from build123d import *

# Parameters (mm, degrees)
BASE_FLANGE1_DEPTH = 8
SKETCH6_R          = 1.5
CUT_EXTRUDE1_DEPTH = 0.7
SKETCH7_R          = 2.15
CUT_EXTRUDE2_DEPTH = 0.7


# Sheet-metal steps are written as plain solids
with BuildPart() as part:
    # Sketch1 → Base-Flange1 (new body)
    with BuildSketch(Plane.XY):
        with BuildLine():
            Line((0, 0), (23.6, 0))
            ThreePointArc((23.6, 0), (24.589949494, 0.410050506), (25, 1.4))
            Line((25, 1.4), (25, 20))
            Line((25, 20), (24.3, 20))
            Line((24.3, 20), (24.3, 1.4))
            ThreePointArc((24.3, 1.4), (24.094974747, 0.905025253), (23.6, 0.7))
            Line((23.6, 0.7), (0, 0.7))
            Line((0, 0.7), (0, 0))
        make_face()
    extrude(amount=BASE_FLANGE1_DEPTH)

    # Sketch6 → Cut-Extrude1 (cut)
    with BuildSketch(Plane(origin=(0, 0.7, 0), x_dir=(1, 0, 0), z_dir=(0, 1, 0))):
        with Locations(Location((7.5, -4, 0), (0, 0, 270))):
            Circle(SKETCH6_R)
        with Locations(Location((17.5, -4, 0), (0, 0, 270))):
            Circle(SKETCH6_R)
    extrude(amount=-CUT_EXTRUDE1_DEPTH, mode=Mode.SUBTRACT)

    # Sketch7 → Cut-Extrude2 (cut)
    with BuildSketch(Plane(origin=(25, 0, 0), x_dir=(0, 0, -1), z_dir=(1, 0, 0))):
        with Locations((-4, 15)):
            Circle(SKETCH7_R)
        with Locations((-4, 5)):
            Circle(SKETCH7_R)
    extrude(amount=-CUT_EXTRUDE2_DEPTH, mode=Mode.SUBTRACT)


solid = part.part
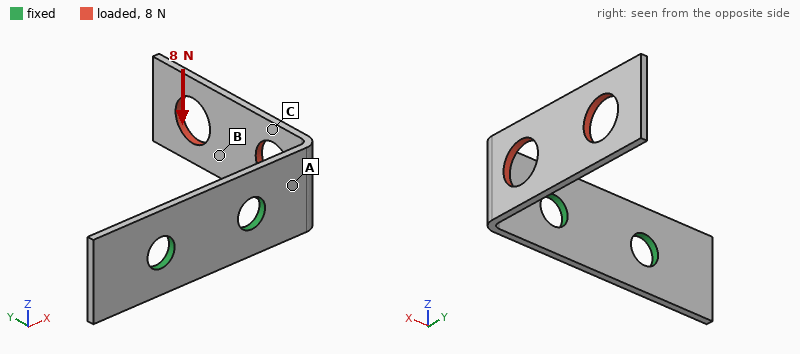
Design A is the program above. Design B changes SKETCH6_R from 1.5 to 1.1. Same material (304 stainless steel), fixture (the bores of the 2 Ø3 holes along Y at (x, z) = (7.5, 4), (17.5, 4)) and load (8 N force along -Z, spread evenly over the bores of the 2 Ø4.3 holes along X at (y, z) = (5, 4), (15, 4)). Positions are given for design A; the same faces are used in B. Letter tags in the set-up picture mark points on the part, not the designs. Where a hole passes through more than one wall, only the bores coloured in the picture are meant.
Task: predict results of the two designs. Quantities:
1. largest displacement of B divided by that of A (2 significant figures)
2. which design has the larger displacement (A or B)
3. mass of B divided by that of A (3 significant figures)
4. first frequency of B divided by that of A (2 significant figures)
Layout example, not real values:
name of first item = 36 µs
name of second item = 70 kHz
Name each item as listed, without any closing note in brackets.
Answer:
largest displacement of B divided by that of A = 1.1
which design has the larger displacement = B
mass of B divided by that of A = 1.02
first frequency of B divided by that of A = 0.98
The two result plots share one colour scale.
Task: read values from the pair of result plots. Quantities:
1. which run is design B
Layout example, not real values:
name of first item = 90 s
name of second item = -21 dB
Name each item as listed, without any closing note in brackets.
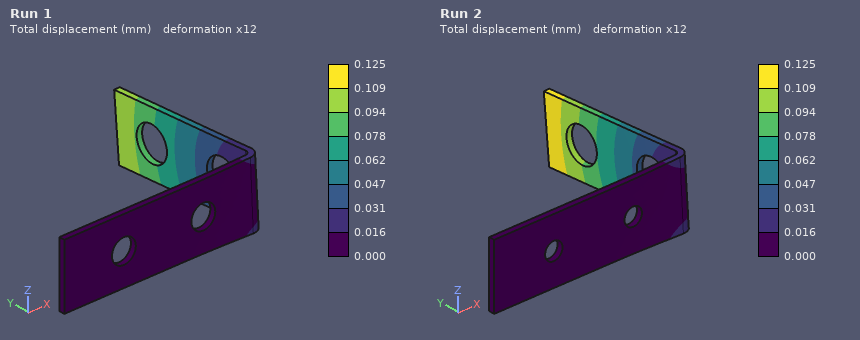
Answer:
which run is design B = Run 2
